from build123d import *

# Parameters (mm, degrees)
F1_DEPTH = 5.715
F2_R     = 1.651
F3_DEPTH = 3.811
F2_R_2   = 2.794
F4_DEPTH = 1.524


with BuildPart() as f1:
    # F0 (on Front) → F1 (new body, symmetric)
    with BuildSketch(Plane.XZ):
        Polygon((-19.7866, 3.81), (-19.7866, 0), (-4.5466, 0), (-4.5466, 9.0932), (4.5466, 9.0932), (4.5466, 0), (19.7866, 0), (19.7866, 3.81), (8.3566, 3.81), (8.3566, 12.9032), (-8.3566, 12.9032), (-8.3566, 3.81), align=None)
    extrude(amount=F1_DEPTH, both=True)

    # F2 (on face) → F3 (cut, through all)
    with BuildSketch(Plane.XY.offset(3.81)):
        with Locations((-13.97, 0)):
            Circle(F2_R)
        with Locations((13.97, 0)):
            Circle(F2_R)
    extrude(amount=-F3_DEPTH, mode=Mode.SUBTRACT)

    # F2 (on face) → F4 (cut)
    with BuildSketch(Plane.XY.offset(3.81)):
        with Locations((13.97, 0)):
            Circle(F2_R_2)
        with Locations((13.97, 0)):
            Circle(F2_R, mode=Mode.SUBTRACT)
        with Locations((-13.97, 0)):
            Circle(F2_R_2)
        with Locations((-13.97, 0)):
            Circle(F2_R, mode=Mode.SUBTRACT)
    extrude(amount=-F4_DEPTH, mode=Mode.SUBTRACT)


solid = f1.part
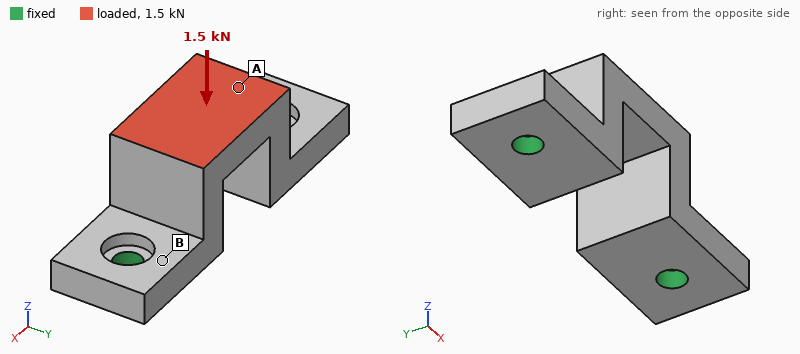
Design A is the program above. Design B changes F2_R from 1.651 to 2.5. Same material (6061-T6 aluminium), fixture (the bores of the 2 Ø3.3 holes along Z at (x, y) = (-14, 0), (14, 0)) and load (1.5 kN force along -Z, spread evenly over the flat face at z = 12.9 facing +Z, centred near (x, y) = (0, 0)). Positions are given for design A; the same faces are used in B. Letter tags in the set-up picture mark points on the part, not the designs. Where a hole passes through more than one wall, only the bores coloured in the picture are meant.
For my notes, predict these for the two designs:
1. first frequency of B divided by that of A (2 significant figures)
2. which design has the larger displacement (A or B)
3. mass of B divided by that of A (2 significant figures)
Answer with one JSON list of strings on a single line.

["1.3", "A", "0.98"]
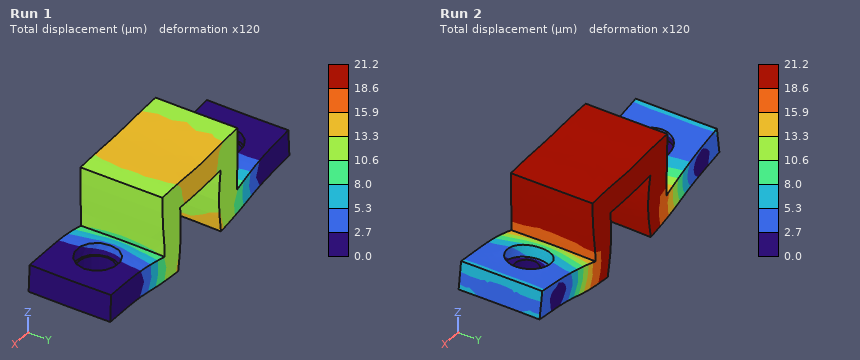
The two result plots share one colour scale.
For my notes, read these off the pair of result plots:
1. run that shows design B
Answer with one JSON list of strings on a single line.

["Run 1"]
